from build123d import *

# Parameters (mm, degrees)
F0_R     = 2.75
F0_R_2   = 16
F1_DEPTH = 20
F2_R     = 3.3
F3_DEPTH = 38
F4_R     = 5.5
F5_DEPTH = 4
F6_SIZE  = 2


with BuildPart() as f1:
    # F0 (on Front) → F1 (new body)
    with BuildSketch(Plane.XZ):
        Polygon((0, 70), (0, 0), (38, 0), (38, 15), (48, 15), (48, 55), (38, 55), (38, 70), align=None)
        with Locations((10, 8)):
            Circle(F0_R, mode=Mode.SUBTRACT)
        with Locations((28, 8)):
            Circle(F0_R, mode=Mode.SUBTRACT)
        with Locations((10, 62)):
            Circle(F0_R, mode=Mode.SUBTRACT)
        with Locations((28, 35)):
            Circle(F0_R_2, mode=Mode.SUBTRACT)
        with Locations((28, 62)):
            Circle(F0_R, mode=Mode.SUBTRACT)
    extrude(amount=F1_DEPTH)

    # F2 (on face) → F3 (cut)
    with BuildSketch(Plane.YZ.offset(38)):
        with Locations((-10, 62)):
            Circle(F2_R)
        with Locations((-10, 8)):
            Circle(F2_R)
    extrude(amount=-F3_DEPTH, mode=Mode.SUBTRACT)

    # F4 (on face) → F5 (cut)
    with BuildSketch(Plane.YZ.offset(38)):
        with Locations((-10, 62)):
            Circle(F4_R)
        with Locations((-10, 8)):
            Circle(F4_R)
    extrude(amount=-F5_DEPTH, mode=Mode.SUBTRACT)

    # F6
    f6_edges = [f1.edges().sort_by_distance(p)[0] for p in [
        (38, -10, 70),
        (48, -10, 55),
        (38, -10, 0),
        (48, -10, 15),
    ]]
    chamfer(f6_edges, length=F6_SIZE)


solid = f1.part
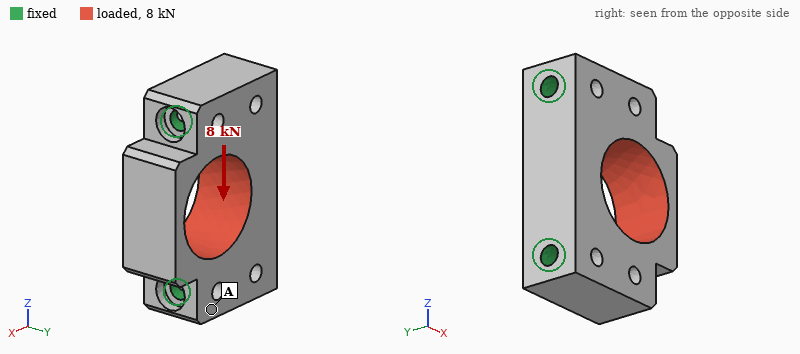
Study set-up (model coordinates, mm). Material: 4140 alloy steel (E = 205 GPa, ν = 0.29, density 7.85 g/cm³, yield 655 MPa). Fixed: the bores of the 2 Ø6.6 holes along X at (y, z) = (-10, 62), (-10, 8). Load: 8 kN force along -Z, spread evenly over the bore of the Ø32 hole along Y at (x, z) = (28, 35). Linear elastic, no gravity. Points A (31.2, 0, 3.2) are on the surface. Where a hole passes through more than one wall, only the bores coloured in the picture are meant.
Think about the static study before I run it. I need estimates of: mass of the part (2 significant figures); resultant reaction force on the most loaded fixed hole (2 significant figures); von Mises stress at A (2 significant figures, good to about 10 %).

320 g
4.0 kN
5.7 MPa
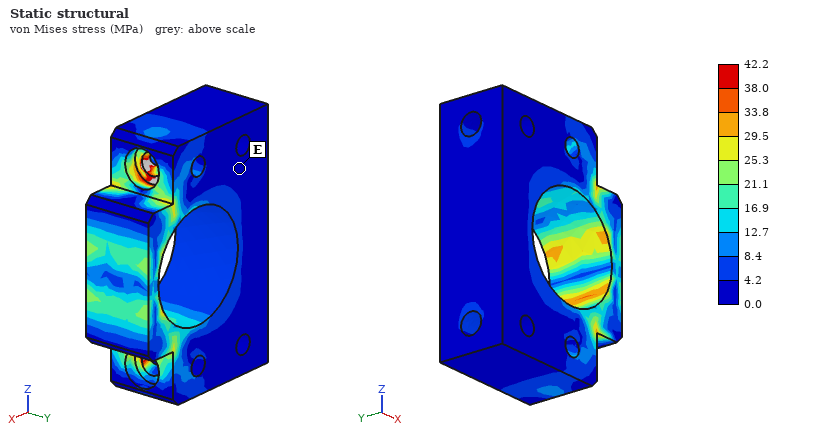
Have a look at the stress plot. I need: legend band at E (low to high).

0.0 to 4.2 MPa
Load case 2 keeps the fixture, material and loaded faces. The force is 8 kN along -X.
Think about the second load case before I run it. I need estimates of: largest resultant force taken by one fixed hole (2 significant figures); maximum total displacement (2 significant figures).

4.1 kN
4.4 µm
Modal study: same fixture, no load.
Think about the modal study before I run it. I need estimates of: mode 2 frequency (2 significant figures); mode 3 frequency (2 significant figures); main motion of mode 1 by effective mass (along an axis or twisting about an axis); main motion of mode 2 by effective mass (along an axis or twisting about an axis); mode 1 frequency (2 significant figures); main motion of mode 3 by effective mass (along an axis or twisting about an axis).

19 kHz
21 kHz
along Y
along Z
14 kHz
along Y
